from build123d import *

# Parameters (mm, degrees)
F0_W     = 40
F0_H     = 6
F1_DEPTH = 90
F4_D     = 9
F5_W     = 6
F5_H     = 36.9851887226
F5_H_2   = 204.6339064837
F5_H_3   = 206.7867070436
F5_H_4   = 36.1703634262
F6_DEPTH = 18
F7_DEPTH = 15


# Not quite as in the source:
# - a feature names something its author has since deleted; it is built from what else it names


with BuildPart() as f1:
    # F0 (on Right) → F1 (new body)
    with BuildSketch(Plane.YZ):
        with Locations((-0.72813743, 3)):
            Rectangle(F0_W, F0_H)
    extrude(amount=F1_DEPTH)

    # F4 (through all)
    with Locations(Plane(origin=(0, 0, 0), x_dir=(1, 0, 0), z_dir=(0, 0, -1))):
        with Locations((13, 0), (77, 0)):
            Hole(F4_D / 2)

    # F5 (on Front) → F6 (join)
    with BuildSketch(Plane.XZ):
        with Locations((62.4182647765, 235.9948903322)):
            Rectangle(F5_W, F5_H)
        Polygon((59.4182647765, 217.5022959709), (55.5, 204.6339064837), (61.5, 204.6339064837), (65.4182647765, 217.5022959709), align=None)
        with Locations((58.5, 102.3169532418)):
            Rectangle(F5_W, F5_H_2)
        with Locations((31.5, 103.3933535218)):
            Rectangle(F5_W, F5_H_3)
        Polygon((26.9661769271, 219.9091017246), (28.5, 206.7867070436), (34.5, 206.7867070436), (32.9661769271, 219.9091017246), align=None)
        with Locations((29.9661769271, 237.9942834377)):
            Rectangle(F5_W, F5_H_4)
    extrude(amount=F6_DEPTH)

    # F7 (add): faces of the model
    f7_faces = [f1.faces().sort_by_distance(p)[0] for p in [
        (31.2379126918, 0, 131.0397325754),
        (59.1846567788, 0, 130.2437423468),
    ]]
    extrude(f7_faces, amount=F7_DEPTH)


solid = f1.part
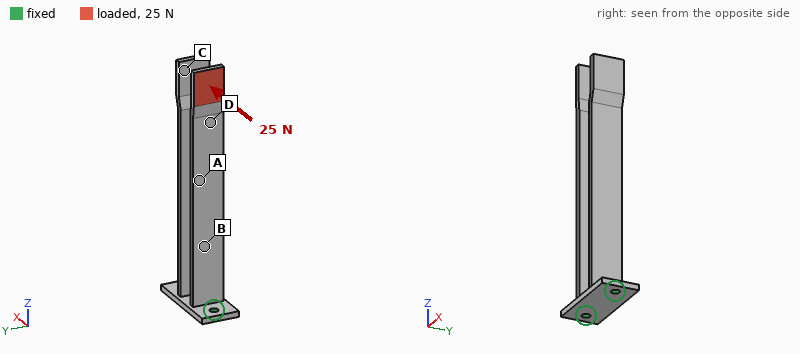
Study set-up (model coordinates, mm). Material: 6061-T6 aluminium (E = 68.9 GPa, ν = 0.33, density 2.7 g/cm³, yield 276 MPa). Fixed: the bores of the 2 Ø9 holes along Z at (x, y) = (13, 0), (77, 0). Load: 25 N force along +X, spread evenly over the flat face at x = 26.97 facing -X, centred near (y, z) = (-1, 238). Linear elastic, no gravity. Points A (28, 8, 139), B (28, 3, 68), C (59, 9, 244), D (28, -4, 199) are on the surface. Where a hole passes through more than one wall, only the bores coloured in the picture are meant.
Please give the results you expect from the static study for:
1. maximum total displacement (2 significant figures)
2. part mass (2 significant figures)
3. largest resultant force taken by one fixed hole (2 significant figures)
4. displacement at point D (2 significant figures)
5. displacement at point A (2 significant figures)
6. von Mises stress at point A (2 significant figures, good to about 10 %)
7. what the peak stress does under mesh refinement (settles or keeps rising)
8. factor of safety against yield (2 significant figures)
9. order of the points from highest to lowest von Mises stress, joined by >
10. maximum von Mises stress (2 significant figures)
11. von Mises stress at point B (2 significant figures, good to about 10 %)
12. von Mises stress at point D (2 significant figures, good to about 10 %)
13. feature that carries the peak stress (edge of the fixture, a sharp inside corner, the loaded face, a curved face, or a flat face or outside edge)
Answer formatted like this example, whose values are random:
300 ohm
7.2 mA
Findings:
3.0 mm
320 g
110 N
2.0 mm
1.1 mm
13 MPa
settles
9.6
B > A > D > C
29 MPa
21 MPa
5.0 MPa
a flat face or outside edge
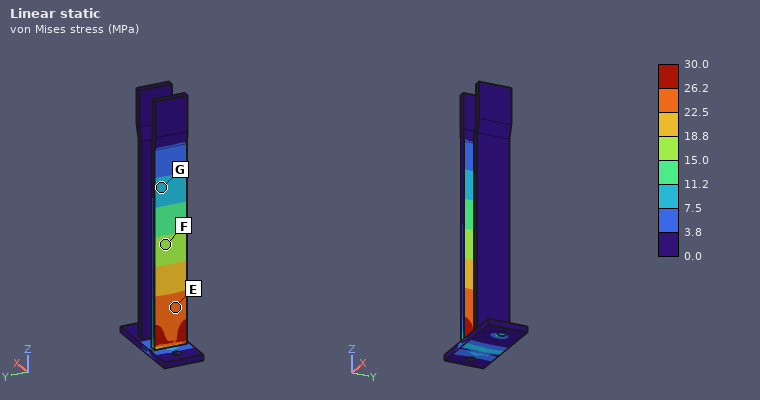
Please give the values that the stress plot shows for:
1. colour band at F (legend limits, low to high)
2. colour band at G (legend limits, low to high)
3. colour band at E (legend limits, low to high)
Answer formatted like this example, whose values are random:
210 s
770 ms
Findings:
15.0 to 18.8 MPa
7.5 to 11.2 MPa
22.5 to 26.2 MPa
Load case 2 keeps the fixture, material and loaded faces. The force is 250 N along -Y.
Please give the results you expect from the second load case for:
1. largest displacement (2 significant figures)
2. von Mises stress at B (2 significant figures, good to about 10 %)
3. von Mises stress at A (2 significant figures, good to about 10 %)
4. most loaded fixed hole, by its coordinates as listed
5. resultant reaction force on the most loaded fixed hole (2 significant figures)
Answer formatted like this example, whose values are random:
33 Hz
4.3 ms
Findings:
2.6 mm
14 MPa
15 MPa
(13, 0)
200 N
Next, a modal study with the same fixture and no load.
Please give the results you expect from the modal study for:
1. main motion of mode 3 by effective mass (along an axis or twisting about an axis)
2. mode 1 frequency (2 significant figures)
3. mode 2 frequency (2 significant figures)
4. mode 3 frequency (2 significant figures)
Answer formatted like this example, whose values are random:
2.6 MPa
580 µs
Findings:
along Y
75 Hz
78 Hz
200 Hz
